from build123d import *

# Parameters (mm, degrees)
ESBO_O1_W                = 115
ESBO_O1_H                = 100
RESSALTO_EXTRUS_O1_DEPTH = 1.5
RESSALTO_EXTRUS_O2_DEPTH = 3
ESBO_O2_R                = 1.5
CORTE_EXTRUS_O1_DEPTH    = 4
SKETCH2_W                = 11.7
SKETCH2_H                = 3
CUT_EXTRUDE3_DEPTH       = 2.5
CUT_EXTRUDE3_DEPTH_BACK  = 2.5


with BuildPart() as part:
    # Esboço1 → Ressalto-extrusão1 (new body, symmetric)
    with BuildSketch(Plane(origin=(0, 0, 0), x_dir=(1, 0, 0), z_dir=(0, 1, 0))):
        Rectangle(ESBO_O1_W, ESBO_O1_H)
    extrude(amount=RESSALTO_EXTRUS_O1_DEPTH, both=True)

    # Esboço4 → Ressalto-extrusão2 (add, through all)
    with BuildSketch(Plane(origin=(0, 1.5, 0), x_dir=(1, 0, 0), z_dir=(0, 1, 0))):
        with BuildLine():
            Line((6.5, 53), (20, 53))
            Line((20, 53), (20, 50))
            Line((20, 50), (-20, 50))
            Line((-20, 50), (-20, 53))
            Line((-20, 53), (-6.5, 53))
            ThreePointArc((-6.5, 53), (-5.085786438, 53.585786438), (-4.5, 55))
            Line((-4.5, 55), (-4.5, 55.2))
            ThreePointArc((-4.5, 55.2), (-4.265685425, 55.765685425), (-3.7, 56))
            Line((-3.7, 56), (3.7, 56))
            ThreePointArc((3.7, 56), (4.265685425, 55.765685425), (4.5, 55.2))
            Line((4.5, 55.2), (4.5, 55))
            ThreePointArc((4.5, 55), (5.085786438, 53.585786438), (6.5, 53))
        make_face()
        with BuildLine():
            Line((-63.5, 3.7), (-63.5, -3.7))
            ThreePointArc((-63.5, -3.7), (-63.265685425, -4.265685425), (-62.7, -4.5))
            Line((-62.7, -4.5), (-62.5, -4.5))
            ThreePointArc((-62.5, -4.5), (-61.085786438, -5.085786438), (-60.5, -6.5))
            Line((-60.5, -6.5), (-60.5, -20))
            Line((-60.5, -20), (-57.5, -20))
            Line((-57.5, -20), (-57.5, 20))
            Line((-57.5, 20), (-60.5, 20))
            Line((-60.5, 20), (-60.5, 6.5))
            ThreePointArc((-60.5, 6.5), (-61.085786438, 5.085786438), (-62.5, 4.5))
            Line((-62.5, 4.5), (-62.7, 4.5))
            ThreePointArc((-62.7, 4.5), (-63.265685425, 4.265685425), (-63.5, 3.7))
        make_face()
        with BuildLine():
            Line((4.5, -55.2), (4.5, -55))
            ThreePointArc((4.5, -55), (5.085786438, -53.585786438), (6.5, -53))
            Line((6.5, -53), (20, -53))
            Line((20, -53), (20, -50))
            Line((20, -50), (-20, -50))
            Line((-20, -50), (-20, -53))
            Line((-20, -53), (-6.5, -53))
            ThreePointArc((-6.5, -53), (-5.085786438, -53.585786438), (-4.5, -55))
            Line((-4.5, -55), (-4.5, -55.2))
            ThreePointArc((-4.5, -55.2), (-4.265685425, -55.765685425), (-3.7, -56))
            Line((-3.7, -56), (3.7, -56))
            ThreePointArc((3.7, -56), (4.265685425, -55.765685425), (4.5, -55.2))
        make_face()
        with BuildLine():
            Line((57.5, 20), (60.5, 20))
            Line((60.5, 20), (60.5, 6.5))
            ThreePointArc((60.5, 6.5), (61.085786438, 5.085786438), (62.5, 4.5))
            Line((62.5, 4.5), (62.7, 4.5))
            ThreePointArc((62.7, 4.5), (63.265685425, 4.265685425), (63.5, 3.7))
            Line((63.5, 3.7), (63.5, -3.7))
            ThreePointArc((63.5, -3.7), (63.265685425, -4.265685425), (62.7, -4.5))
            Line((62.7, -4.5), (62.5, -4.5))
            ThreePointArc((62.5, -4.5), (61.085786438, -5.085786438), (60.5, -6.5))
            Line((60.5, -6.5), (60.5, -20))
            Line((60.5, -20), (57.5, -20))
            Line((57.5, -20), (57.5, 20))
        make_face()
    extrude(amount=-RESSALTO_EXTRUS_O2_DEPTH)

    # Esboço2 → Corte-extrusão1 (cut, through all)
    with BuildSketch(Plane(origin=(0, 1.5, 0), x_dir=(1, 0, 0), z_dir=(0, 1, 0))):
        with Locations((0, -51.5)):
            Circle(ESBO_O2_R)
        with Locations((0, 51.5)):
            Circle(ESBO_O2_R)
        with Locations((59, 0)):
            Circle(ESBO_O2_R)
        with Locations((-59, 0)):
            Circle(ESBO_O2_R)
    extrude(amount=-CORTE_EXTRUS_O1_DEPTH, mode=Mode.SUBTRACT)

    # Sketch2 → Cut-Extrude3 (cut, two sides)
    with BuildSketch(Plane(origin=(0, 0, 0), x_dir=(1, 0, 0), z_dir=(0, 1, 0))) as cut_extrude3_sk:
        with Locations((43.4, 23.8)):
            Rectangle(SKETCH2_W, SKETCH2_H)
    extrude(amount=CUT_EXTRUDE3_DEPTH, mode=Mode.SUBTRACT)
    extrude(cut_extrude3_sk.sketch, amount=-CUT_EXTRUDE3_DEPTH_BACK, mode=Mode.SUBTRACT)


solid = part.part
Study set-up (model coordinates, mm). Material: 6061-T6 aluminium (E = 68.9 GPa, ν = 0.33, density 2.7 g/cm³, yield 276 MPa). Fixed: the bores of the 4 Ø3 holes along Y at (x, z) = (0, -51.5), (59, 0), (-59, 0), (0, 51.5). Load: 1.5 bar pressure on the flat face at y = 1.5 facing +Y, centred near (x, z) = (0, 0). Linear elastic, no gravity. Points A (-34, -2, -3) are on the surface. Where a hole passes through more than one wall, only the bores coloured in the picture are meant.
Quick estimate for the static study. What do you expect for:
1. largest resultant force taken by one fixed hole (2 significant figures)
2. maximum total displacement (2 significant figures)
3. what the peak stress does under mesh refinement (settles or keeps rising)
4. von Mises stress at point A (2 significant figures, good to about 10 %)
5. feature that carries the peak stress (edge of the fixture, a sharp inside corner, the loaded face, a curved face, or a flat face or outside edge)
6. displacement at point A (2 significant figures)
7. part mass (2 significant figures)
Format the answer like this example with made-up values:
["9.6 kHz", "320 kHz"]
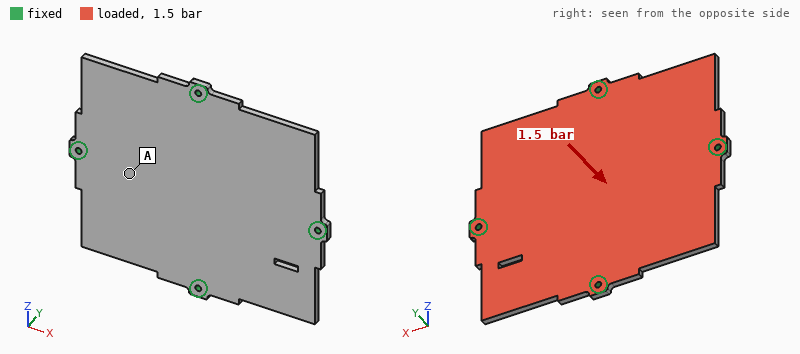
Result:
["460 N", "0.24 mm", "keeps rising", "20 MPa", "edge of the fixture", "0.15 mm", "97 g"]
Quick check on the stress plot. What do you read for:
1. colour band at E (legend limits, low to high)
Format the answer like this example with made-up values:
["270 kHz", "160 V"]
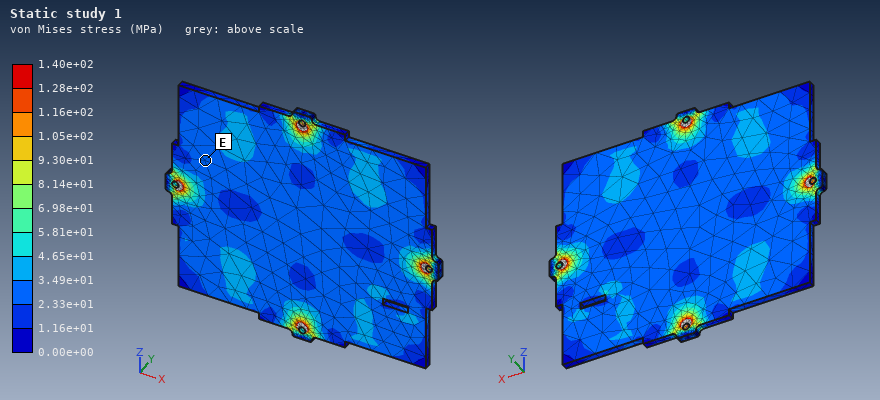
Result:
["2.33e+01 to 3.49e+01 MPa"]
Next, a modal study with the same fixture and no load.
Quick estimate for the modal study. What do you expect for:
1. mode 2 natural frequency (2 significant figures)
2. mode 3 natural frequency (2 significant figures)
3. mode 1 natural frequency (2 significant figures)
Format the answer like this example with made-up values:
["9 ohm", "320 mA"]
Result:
["1600 Hz", "1700 Hz", "1500 Hz"]
